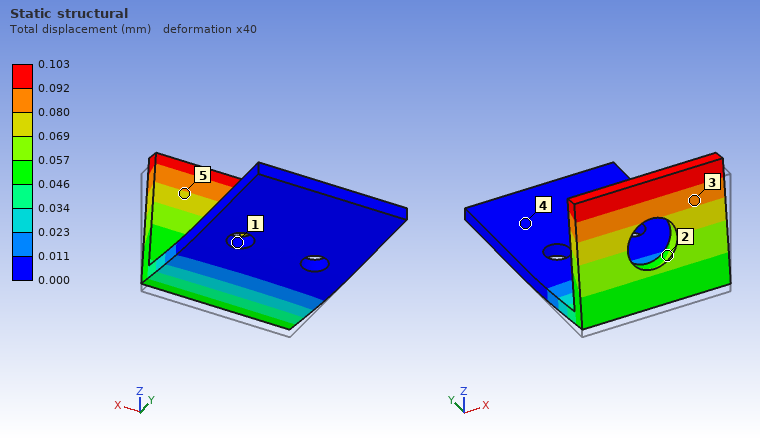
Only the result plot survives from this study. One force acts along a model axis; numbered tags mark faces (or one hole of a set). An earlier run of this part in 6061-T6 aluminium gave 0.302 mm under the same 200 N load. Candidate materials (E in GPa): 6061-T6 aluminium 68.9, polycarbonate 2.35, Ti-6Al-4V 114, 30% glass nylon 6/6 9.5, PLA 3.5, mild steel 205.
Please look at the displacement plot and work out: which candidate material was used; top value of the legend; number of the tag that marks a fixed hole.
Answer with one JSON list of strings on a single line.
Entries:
["mild steel", "0.103 mm", "1"]
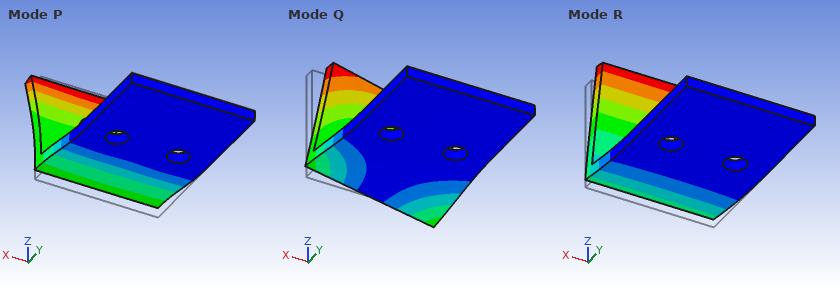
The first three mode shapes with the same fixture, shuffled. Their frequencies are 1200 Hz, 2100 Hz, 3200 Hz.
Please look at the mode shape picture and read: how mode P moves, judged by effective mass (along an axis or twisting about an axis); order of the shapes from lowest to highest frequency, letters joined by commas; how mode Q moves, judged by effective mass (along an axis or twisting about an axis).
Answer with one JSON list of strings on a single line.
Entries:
["along Z", "R, Q, P", "along X"]
